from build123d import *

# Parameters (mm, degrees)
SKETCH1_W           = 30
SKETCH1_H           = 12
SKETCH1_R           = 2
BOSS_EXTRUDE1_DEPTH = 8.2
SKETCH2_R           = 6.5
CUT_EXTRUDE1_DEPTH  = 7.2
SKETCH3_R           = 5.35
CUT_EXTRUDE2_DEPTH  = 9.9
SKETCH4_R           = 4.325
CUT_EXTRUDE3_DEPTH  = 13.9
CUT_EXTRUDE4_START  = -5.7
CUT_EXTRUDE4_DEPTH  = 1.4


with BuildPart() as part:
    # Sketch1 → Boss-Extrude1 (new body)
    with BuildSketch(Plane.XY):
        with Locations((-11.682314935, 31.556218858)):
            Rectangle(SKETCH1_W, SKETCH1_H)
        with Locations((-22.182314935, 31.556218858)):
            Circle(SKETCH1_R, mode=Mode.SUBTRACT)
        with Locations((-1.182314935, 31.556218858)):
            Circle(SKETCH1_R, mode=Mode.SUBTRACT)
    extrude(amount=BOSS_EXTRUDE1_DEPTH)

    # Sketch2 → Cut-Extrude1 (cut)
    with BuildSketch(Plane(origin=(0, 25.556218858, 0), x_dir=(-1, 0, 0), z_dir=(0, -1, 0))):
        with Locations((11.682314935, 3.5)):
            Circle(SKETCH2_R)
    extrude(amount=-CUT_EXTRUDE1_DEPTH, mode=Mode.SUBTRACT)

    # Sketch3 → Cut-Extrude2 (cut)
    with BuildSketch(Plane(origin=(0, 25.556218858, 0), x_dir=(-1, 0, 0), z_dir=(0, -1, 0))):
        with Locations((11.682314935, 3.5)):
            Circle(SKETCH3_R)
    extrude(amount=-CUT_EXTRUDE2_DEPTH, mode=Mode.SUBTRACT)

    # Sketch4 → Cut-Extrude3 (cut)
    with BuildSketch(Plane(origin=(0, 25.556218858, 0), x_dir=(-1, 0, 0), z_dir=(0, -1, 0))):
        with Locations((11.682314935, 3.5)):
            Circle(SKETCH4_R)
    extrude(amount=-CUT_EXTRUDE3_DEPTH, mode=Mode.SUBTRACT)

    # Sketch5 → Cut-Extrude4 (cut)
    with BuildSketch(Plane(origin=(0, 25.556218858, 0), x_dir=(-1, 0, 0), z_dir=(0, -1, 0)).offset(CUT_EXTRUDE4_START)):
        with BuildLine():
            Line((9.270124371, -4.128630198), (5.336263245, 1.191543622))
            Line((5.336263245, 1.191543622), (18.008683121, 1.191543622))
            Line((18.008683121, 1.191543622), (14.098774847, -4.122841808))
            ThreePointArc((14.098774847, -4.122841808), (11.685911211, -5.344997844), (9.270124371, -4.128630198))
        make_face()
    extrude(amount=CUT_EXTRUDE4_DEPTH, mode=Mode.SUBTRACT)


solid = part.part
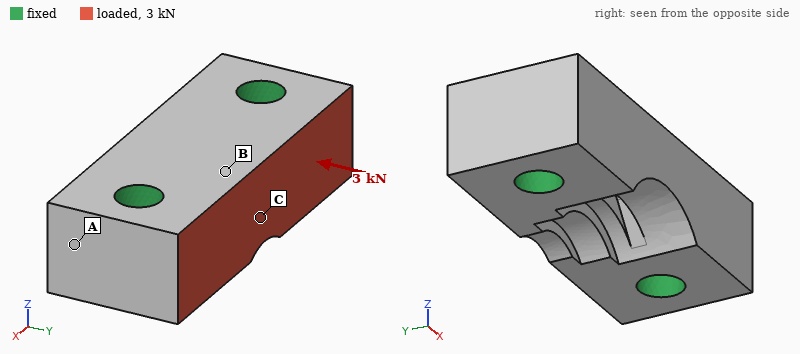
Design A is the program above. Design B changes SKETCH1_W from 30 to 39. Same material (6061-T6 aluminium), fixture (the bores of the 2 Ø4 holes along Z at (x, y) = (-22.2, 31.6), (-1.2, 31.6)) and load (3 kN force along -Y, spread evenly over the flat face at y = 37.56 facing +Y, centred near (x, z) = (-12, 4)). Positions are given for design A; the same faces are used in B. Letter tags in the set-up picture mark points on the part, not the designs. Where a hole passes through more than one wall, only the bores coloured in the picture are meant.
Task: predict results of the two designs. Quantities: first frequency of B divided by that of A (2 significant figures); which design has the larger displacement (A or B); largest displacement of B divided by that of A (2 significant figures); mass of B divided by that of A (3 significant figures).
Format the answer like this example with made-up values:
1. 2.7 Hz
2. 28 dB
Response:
1. 0.82
2. A
3. 0.69
4. 1.35
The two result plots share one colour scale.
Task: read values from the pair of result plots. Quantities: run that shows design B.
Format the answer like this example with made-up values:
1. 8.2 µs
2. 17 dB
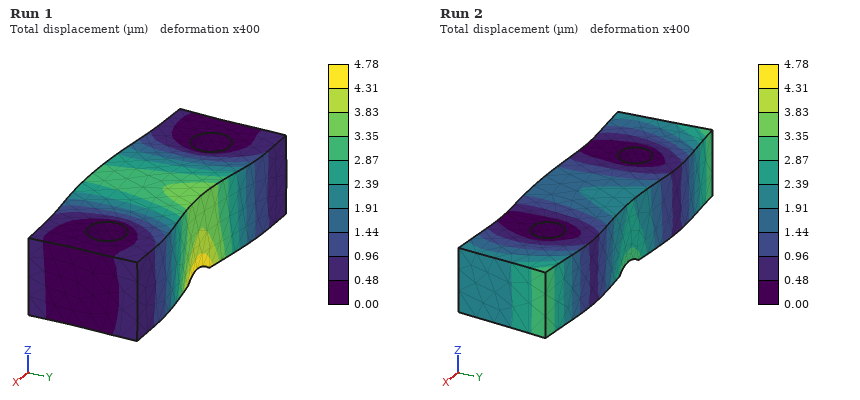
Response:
1. Run 2
